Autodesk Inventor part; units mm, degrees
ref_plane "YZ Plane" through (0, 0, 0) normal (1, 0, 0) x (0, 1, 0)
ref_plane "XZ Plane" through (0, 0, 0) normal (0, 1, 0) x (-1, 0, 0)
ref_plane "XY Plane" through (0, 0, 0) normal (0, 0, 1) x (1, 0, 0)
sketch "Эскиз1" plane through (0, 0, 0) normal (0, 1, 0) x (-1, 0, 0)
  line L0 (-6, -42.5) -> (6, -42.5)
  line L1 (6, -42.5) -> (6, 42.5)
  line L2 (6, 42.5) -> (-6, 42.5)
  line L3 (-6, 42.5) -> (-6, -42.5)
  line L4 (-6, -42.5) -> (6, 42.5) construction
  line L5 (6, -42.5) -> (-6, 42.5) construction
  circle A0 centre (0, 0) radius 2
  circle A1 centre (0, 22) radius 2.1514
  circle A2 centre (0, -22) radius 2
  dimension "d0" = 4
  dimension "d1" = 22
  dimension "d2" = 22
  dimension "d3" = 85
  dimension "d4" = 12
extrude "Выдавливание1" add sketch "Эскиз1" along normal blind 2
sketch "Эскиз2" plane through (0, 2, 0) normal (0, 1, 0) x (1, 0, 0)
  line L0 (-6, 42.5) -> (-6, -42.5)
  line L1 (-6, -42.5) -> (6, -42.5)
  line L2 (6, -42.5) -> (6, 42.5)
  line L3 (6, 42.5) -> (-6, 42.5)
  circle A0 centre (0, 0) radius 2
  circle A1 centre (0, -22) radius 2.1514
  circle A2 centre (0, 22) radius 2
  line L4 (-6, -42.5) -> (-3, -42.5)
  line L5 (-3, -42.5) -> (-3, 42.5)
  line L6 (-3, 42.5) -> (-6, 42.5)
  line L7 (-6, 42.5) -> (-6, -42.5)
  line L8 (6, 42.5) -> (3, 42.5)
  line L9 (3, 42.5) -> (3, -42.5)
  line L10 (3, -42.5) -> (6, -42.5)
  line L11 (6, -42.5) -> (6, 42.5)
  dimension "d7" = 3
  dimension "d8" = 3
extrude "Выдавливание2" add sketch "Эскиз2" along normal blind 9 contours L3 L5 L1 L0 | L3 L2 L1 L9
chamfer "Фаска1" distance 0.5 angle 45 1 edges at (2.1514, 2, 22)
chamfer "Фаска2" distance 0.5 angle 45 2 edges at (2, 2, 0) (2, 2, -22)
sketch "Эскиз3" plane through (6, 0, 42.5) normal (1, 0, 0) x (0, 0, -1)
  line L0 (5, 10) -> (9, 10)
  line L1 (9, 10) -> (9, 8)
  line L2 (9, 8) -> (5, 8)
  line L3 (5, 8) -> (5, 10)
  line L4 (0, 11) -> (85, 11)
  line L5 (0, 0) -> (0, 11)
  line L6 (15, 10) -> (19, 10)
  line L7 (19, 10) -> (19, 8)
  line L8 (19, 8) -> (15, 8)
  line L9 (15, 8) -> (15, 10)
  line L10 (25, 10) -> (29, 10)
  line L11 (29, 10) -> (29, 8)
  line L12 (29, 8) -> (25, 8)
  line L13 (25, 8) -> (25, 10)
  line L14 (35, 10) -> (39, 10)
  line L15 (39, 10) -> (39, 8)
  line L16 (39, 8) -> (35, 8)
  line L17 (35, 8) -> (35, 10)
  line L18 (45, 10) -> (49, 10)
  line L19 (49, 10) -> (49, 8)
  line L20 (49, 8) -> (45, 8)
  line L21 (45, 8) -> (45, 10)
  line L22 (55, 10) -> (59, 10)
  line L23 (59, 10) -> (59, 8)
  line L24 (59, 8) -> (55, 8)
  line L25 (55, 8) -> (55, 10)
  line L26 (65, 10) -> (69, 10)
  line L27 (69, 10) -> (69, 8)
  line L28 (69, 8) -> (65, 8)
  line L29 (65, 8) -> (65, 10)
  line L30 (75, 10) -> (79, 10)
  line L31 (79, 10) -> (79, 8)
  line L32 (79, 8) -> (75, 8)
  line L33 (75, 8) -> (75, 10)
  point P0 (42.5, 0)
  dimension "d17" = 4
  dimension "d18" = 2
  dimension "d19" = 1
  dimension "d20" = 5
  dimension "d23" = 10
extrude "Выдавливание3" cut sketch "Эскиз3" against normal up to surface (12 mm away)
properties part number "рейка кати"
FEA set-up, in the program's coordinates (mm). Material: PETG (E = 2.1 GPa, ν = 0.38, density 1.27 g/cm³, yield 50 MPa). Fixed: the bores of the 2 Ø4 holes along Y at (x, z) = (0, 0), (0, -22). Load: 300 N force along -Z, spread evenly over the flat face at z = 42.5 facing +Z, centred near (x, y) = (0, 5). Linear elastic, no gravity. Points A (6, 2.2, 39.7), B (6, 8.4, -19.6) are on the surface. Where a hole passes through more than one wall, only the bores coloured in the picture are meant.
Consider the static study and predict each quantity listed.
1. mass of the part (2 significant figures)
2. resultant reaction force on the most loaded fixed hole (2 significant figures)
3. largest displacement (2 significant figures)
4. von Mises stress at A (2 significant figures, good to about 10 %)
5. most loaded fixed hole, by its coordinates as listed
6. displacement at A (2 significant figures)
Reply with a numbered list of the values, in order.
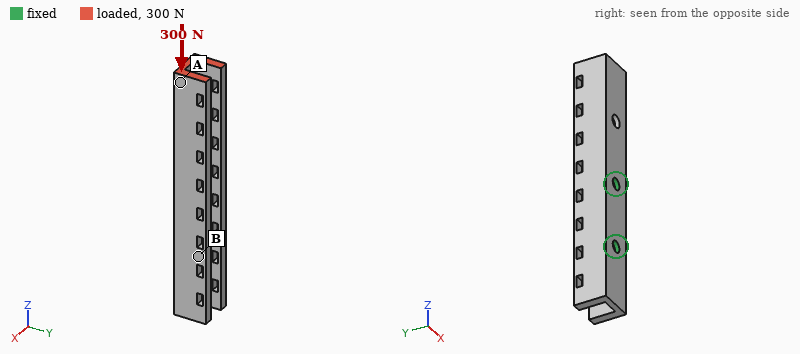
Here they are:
1. 7.8 g
2. 200 N
3. 0.37 mm
4. 3.9 MPa
5. (0, 0)
6. 0.31 mm
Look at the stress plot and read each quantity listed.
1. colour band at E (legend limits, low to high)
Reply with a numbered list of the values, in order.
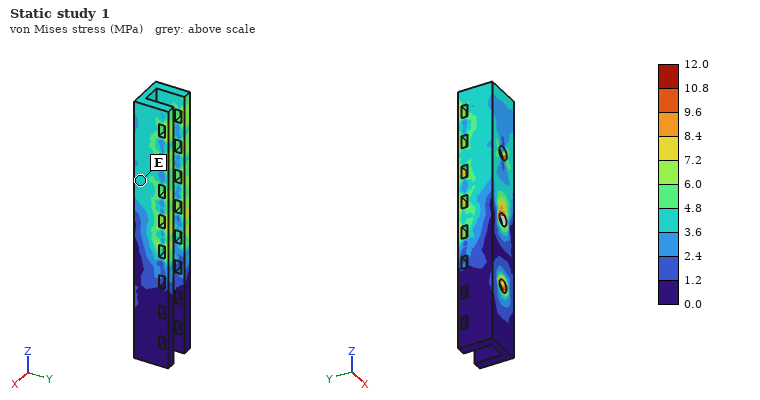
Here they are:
1. 3.6 to 4.8 MPa
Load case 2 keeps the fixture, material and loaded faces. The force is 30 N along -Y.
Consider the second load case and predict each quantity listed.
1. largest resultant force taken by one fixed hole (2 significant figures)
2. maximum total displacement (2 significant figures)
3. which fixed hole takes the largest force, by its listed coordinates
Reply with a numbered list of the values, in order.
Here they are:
1. 110 N
2. 0.86 mm
3. (0, 0)
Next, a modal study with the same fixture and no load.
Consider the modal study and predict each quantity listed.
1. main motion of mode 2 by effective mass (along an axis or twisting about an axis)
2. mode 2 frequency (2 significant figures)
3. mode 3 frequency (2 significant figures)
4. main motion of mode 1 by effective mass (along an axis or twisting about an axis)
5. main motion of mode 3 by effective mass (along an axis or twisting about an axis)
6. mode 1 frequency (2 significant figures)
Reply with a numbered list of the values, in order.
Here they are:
1. along Y
2. 880 Hz
3. 1600 Hz
4. along X
5. twisting about Z
6. 760 Hz
